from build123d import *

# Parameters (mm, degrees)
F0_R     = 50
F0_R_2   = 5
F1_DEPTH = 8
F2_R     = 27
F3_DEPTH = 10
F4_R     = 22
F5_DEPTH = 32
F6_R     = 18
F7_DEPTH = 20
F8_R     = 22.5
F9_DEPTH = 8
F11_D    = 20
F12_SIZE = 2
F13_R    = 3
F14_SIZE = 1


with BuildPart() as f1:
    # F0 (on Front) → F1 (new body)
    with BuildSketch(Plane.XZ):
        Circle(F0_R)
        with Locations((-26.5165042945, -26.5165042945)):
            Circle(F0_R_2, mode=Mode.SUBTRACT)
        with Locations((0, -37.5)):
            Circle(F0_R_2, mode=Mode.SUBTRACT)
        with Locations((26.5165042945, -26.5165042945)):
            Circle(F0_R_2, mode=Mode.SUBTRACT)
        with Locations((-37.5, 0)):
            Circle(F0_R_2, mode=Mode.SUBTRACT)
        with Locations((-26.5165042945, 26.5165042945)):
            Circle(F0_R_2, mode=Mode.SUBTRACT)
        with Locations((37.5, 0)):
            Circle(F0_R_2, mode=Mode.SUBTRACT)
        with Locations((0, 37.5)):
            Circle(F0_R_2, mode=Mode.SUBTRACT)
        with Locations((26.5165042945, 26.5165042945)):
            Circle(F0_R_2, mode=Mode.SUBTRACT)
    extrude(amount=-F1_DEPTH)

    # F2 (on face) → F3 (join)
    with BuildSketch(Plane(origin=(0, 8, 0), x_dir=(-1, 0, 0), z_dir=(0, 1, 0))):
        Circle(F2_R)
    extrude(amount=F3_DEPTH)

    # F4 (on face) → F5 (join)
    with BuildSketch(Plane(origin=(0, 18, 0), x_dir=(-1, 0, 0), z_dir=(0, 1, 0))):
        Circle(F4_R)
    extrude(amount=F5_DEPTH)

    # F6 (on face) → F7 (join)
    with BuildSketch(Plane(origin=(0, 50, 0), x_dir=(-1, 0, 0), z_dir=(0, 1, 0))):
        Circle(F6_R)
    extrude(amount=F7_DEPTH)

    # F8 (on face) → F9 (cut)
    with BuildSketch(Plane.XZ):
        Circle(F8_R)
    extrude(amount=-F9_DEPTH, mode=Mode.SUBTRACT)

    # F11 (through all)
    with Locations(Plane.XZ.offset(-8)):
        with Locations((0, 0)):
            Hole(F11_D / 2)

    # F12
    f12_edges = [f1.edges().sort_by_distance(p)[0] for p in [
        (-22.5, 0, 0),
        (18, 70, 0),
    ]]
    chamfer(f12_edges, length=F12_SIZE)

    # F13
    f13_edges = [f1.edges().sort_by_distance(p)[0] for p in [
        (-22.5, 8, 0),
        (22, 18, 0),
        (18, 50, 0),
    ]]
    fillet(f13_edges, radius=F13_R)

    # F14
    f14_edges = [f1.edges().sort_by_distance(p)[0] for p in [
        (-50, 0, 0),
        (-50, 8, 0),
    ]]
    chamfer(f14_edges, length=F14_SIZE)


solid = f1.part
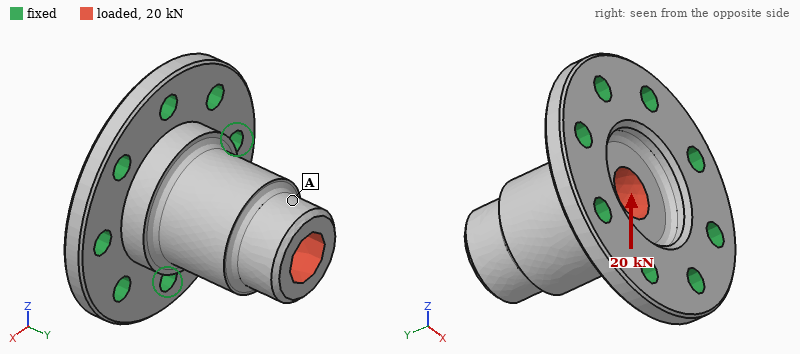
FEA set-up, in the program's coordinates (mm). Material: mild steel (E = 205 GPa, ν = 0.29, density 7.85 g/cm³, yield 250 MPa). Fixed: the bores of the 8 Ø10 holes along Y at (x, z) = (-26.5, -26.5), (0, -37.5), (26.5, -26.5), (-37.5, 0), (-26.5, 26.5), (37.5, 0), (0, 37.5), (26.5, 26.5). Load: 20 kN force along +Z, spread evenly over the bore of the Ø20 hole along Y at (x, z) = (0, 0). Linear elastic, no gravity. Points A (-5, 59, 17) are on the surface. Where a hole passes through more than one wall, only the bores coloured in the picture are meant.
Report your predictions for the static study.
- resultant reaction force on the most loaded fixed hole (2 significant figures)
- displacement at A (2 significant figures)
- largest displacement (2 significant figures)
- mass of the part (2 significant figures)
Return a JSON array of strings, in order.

["7.5 kN", "36 µm", "43 µm", "920 g"]
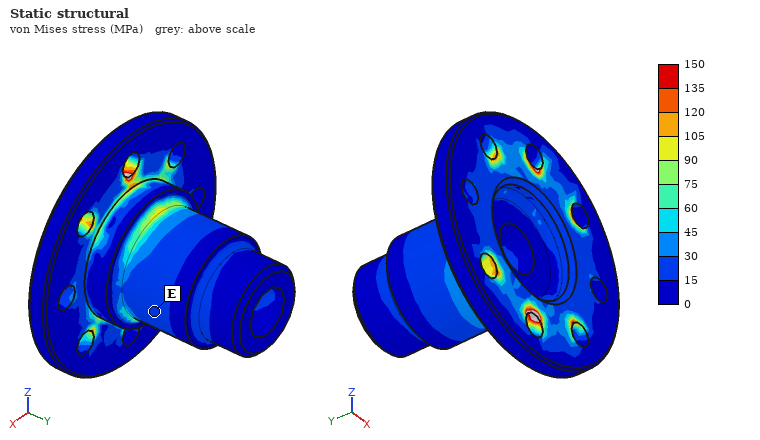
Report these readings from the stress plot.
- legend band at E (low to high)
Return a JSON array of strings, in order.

["15 to 30 MPa"]
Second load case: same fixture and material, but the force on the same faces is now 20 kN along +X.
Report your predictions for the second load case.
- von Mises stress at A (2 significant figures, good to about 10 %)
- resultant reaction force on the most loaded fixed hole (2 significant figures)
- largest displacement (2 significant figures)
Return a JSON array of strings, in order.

["13 MPa", "7.5 kN", "43 µm"]
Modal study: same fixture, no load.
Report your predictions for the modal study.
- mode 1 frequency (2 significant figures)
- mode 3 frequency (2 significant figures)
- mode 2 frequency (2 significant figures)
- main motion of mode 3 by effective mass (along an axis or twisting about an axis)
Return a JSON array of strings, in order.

["6300 Hz", "12 kHz", "6300 Hz", "along Y"]
